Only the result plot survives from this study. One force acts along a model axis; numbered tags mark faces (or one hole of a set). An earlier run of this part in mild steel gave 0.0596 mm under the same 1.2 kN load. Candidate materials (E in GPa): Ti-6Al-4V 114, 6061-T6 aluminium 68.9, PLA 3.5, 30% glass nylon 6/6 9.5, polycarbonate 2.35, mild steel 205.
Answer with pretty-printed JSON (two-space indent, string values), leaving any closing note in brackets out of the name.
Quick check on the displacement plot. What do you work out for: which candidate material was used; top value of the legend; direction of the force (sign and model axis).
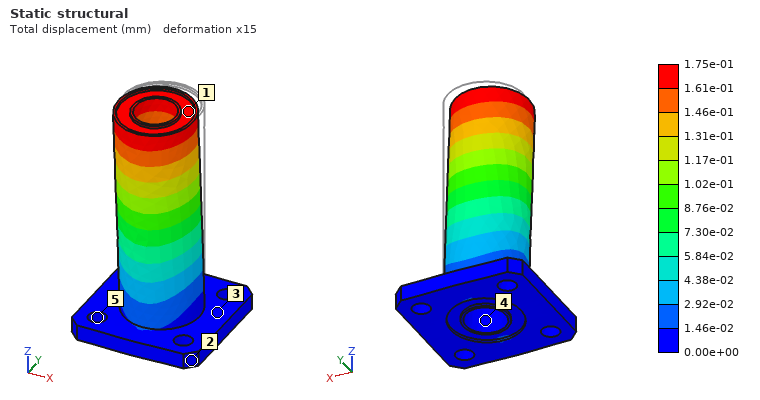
{
  "which candidate material was used": "6061-T6 aluminium",
  "top value of the legend": "1.75e-01 mm",
  "direction of the force": "-Y"
}
